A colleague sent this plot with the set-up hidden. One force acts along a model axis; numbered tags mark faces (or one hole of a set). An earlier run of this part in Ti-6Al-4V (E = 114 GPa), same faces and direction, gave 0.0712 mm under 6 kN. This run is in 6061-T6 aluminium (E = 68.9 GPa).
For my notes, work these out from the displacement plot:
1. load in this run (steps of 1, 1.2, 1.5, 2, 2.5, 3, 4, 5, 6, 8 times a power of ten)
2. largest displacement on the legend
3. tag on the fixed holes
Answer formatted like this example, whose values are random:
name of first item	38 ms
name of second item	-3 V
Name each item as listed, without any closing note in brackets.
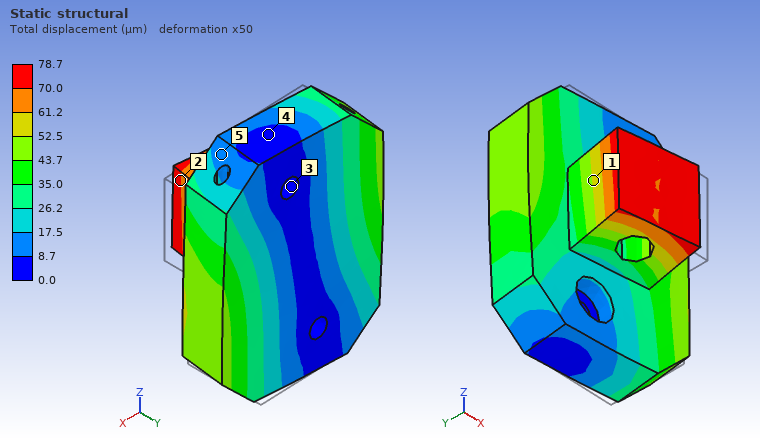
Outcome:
load in this run	4 kN
largest displacement on the legend	78.7 µm
tag on the fixed holes	3
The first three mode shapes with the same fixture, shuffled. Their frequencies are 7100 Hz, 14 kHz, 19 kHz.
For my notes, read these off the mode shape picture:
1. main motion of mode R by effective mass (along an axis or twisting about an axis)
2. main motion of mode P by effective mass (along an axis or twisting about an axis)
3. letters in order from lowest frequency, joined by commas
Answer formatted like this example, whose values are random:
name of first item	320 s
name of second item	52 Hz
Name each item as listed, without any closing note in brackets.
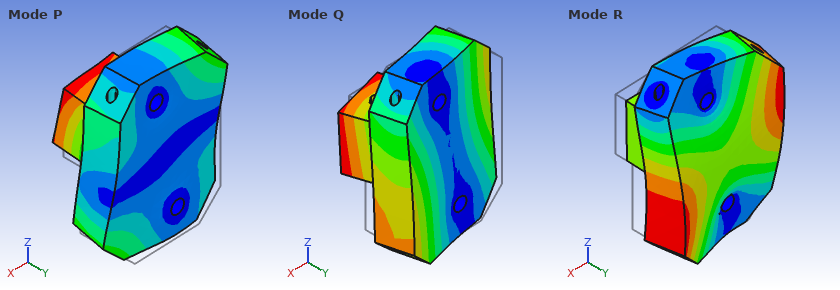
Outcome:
main motion of mode R by effective mass	along Y
main motion of mode P by effective mass	along Z
letters in order from lowest frequency, joined by commas	Q, R, P
